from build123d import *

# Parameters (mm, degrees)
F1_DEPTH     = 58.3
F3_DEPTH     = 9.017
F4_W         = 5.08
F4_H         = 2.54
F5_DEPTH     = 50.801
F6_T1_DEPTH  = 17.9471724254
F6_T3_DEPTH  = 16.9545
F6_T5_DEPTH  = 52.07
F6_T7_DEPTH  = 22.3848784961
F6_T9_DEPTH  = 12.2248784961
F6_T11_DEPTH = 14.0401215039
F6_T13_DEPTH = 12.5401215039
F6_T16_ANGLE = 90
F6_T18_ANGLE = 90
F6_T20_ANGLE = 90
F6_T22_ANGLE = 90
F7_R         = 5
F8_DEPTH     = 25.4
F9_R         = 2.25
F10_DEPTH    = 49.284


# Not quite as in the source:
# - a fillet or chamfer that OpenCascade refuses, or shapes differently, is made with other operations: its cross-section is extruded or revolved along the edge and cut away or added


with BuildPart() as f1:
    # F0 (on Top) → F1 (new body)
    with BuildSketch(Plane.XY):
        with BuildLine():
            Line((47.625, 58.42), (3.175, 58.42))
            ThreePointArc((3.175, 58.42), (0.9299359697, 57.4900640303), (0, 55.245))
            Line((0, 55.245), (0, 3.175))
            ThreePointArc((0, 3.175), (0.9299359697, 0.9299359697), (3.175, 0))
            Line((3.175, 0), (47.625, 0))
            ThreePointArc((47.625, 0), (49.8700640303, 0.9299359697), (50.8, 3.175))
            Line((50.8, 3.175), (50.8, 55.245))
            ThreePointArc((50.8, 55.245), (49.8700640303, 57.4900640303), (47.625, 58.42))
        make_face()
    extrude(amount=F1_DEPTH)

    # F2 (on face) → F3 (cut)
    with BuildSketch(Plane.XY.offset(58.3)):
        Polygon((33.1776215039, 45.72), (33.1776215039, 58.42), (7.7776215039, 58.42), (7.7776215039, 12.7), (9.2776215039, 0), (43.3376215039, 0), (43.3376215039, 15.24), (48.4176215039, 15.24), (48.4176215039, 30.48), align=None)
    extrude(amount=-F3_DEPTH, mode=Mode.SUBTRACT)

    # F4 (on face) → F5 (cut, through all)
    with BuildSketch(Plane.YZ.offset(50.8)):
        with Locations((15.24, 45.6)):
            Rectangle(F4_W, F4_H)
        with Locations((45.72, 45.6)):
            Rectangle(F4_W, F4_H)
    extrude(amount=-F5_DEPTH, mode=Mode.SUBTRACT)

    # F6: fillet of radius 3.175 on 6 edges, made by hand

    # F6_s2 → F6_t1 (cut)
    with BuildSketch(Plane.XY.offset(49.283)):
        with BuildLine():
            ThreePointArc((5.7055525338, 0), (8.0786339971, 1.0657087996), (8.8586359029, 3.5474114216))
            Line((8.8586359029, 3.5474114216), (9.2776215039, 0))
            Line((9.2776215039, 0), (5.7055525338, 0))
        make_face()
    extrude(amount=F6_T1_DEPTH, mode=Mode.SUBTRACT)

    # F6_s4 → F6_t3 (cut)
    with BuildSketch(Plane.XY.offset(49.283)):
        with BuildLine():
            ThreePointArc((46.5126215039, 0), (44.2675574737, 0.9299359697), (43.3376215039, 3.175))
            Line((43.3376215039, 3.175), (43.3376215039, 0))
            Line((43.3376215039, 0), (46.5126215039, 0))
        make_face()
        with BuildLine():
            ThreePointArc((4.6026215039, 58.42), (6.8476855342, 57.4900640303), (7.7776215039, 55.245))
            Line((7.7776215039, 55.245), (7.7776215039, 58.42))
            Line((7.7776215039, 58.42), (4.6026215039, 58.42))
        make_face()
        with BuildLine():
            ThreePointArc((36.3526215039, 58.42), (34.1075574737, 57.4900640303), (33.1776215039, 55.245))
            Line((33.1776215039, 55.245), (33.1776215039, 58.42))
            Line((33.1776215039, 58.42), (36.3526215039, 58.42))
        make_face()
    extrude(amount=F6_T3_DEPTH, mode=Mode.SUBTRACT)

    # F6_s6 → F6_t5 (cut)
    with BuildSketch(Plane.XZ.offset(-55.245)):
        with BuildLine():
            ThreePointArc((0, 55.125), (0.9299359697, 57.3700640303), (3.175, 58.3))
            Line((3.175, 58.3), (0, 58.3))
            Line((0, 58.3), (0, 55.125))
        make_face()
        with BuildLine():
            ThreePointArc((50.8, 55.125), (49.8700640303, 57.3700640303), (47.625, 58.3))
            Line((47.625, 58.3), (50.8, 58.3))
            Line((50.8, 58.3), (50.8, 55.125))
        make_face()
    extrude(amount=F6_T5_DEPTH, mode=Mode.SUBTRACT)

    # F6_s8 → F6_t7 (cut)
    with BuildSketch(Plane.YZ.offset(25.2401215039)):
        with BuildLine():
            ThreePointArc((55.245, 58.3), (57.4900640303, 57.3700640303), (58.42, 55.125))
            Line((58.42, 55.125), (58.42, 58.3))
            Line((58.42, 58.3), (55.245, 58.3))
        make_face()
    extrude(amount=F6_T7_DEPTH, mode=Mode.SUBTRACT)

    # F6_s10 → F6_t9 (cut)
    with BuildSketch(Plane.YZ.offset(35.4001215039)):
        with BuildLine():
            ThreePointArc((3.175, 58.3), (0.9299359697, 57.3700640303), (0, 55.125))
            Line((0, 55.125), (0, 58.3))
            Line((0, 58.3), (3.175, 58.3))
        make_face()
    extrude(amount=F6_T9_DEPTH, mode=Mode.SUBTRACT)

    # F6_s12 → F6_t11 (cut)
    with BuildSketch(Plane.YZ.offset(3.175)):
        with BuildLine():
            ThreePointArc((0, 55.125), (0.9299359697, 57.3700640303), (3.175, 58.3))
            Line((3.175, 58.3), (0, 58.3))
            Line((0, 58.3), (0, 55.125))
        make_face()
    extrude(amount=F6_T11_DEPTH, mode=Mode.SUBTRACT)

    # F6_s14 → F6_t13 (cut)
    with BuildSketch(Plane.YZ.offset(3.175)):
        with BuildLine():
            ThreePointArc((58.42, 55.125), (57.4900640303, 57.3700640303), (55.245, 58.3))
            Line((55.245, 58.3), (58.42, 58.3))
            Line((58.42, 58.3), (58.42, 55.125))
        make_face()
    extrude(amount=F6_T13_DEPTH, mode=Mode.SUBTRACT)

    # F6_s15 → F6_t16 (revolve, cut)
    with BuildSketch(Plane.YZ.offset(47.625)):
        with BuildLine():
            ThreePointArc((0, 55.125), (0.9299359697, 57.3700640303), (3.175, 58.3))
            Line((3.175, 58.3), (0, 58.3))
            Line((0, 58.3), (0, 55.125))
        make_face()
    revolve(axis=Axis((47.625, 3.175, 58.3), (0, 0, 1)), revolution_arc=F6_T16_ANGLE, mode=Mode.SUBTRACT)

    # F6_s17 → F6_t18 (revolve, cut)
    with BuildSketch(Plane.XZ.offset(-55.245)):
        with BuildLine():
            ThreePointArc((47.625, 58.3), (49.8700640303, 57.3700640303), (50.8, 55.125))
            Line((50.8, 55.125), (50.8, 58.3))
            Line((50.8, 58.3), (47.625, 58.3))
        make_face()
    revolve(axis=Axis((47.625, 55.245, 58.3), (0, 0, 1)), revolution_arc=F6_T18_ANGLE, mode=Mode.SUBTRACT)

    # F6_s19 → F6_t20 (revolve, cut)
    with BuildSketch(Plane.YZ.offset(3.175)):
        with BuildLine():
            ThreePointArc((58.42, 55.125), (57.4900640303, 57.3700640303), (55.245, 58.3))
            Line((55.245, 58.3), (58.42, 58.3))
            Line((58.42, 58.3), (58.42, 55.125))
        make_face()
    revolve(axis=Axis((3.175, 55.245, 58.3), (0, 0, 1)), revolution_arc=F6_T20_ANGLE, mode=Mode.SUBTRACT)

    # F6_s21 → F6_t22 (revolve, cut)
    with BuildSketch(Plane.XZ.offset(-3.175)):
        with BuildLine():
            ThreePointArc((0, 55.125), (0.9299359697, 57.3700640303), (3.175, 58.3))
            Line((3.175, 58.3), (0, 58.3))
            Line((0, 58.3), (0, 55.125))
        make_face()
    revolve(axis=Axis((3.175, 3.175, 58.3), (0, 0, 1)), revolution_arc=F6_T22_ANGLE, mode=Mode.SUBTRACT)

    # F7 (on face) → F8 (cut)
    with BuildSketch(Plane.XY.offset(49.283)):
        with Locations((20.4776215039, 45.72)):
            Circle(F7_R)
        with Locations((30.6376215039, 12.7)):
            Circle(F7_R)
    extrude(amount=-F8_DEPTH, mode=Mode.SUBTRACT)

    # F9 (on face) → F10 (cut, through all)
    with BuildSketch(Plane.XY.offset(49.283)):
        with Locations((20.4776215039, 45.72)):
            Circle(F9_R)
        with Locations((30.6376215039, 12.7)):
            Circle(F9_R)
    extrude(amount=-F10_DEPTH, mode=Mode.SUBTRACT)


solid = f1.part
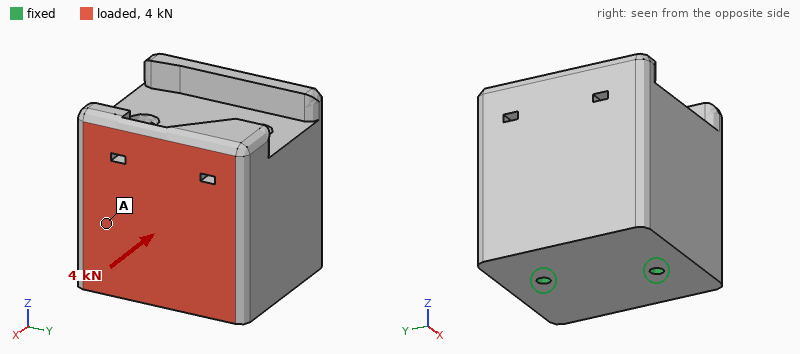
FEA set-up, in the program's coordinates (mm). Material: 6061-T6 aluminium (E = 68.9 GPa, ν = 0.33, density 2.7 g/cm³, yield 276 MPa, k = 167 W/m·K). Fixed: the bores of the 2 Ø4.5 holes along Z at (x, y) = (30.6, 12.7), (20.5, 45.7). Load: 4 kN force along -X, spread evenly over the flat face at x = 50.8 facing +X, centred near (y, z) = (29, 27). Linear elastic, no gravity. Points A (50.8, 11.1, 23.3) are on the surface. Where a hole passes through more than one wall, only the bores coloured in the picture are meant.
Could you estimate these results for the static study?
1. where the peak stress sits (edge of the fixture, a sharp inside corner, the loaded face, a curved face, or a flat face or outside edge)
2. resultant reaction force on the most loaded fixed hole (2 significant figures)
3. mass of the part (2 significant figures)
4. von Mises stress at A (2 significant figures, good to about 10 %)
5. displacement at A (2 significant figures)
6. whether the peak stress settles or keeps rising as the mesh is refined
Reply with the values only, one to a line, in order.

edge of the fixture
2.1 kN
400 g
3.7 MPa
3.9 µm
keeps rising
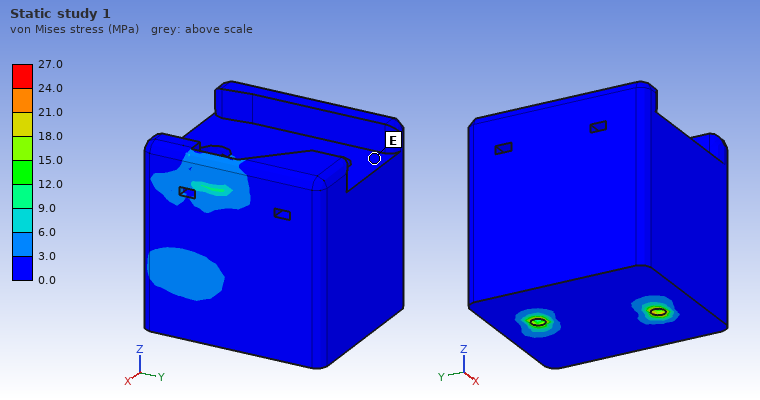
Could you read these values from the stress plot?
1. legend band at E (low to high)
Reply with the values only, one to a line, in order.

0.0 to 3.0 MPa
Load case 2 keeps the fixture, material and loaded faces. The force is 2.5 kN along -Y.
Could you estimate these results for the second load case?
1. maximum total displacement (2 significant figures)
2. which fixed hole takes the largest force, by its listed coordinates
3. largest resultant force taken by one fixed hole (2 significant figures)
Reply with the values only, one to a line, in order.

5.5 µm
(30.6, 12.7)
2.5 kN
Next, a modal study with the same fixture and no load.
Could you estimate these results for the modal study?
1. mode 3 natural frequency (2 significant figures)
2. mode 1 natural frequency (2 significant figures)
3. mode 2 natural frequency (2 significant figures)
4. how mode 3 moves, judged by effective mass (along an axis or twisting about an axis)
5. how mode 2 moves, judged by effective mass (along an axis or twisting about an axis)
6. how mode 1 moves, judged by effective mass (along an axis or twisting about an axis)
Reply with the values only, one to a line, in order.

12 kHz
5900 Hz
10 kHz
twisting about Z
along Y
along X
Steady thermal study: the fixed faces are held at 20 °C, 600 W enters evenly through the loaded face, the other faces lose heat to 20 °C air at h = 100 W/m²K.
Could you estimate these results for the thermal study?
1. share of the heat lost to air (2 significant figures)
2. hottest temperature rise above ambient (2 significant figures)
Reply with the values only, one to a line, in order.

8.1 %
67 K
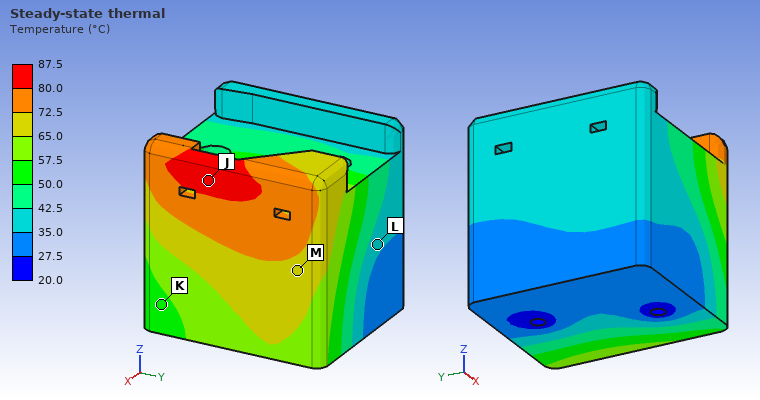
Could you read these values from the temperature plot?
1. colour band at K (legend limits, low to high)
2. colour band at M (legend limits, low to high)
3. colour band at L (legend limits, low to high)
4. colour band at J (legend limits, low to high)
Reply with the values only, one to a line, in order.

50.0 to 57.5 °C
65.0 to 72.5 °C
35.0 to 42.5 °C
80.0 to 87.5 °C
